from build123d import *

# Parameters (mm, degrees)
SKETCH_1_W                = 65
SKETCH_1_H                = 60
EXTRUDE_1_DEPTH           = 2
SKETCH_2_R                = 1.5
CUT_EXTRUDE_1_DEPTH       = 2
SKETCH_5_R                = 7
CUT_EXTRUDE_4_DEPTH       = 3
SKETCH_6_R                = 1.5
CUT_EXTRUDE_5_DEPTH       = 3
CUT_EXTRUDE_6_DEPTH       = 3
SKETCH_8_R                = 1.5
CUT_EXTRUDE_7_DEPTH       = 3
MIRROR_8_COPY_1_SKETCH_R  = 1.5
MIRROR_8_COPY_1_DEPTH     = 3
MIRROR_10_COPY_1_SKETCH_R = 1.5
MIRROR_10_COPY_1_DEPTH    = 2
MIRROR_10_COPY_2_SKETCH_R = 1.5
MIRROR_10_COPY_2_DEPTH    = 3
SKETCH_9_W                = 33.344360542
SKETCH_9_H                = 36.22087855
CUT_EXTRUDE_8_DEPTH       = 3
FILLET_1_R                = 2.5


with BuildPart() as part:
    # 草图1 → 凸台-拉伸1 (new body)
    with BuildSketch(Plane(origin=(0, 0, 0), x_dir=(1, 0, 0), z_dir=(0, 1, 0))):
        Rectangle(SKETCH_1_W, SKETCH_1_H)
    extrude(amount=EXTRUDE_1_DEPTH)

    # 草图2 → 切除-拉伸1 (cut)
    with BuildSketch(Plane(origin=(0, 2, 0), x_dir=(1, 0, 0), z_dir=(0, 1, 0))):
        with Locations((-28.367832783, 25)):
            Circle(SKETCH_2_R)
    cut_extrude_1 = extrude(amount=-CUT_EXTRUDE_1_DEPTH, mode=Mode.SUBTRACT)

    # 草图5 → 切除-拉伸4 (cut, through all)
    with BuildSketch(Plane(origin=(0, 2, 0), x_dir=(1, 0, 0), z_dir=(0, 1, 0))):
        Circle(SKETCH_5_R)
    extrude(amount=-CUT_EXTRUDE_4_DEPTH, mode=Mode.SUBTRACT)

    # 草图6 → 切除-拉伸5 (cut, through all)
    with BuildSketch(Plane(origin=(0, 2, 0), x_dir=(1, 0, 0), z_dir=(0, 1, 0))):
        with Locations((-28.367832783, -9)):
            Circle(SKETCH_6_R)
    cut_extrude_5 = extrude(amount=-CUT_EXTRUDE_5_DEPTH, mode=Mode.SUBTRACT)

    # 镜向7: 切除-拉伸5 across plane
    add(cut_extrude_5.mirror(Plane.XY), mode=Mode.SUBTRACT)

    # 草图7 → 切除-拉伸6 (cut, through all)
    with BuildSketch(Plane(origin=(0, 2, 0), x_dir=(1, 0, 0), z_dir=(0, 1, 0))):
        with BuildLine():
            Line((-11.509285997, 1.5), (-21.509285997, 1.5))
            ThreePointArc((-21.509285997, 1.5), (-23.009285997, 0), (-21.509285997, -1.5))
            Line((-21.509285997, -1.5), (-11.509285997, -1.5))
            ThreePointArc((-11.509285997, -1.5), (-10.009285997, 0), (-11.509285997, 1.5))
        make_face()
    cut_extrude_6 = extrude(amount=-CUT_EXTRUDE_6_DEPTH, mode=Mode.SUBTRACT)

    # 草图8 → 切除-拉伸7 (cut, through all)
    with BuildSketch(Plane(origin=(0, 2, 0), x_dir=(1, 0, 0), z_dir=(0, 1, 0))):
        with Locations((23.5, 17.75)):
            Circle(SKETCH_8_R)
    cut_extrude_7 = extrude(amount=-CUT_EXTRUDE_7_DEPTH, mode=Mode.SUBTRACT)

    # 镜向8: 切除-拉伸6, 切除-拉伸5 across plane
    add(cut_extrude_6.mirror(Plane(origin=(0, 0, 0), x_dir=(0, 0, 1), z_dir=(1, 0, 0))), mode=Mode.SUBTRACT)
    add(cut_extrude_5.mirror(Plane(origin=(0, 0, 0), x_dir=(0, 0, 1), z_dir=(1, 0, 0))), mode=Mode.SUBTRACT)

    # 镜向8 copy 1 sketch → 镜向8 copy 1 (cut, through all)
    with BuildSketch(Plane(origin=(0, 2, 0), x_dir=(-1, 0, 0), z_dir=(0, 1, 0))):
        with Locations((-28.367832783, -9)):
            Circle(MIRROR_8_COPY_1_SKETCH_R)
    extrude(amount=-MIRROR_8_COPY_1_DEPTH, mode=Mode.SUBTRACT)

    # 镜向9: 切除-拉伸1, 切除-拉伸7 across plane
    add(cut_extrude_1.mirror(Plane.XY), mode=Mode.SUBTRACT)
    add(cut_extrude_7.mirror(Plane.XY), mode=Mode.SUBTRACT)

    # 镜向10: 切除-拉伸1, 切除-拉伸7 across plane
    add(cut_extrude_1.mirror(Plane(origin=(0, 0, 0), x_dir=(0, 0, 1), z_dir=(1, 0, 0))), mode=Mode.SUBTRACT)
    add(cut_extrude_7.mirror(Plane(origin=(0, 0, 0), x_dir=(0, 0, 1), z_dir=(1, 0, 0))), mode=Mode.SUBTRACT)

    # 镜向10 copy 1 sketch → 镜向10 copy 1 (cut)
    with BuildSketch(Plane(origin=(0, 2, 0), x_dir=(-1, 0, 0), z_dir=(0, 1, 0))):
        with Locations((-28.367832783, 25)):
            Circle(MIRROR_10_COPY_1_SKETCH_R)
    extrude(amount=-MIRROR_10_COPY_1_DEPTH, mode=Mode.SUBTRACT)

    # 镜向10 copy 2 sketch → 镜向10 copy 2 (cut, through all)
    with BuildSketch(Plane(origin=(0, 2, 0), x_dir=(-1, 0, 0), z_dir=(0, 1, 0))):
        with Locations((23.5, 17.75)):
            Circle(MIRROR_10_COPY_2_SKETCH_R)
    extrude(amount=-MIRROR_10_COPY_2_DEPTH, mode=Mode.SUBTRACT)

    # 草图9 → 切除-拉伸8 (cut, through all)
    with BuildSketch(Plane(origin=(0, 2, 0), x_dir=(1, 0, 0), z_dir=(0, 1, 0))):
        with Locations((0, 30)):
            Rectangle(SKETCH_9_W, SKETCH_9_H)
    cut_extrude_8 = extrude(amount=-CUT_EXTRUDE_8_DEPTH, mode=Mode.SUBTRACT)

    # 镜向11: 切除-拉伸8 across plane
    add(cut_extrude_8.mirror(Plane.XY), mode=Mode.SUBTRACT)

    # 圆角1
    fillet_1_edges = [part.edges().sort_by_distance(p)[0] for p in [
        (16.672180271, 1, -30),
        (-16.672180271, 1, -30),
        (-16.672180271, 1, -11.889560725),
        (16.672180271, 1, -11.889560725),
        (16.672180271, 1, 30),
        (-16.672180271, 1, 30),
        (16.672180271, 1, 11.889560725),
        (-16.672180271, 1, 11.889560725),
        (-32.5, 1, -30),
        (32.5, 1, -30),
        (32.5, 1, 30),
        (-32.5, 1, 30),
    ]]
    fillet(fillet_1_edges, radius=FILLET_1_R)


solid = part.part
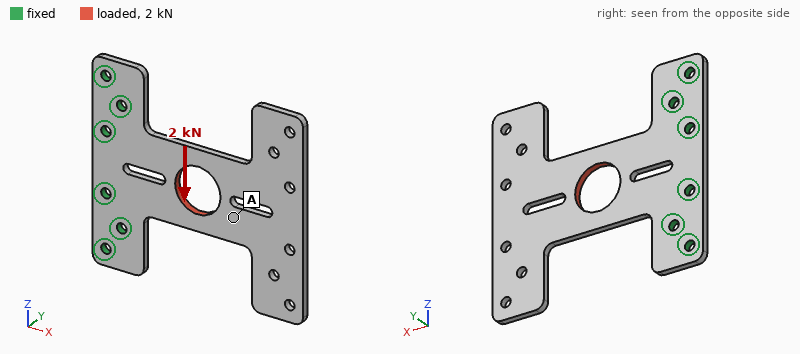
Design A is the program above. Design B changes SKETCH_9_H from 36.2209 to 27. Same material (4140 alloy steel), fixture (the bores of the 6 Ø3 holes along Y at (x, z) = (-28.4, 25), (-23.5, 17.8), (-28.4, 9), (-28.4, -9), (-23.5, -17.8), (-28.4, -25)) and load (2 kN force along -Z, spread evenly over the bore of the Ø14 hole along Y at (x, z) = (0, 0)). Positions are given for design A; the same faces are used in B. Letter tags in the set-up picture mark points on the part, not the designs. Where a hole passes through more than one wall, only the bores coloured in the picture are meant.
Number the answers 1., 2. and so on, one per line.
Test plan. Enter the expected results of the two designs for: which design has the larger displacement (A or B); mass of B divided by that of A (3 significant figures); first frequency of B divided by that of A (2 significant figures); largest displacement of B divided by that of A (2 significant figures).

1. A
2. 1.13
3. 1.2
4. 0.41
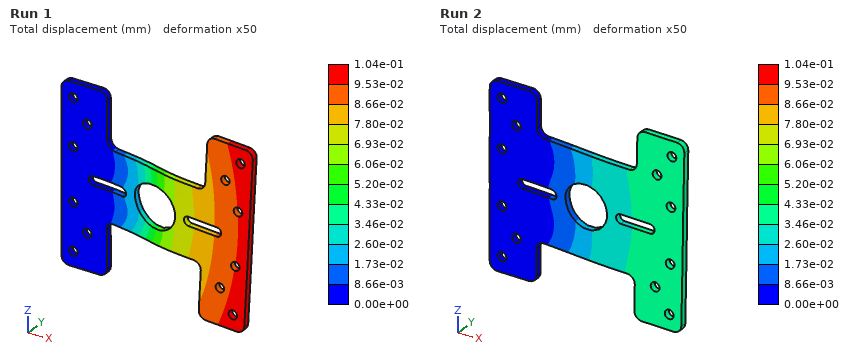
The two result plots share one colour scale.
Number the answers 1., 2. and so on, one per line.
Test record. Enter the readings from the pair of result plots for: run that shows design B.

1. Run 2
